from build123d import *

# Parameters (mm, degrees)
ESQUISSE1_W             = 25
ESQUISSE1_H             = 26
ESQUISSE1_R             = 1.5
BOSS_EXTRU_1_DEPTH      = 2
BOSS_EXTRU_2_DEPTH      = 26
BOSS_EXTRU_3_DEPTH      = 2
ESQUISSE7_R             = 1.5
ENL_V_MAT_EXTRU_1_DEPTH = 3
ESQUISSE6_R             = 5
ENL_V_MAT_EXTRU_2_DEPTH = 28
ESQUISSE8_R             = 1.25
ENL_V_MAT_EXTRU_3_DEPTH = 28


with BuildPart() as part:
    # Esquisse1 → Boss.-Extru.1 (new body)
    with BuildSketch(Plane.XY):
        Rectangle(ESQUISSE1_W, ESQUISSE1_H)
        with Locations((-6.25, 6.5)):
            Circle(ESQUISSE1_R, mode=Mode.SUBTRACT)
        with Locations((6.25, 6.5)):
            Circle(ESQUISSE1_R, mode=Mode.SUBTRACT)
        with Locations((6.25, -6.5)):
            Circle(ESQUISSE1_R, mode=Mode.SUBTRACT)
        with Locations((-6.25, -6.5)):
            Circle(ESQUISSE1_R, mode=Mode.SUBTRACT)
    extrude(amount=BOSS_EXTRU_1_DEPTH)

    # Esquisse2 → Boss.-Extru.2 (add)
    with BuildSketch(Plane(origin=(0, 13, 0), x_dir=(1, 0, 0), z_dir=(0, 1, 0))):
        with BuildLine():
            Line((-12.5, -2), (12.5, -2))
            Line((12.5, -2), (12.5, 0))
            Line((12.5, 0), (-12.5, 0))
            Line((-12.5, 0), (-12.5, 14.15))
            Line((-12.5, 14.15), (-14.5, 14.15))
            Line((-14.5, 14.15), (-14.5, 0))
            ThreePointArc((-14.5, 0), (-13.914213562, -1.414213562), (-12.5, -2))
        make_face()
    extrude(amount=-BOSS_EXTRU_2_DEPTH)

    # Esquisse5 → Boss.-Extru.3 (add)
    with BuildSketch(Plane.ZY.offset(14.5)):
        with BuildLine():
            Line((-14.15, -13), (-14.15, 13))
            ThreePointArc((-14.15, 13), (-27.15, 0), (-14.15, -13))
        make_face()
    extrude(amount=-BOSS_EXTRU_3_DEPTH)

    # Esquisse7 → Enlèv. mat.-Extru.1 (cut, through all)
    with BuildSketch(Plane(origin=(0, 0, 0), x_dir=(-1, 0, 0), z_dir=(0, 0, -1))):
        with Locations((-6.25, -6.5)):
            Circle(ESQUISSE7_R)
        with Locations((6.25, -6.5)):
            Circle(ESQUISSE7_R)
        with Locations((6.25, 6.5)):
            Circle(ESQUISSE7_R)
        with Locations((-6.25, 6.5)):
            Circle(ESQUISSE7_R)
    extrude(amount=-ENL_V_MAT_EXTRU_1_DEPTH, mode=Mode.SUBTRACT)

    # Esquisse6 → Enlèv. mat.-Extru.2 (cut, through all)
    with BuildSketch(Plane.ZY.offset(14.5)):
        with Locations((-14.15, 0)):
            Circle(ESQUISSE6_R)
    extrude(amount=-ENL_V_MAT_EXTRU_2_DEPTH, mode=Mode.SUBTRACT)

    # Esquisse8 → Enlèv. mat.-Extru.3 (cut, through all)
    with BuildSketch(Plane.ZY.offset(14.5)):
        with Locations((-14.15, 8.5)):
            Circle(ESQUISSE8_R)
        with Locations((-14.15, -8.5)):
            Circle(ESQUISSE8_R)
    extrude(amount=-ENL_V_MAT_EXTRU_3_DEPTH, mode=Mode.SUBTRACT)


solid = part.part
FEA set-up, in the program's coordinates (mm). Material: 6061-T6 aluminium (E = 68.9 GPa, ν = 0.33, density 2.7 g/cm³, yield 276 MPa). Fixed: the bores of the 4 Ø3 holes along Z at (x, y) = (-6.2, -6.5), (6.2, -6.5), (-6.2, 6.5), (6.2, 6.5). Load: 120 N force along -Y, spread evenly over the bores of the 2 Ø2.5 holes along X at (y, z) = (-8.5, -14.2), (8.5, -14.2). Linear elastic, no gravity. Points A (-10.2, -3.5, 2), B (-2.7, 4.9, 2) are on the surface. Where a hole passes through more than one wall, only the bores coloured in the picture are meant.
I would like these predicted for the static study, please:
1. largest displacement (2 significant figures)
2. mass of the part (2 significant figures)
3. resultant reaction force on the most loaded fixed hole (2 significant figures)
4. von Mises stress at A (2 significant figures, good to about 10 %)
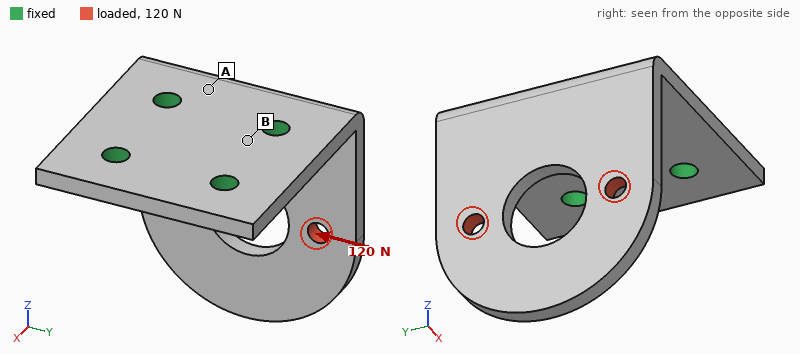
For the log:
55 µm
6.5 g
140 N
23 MPa
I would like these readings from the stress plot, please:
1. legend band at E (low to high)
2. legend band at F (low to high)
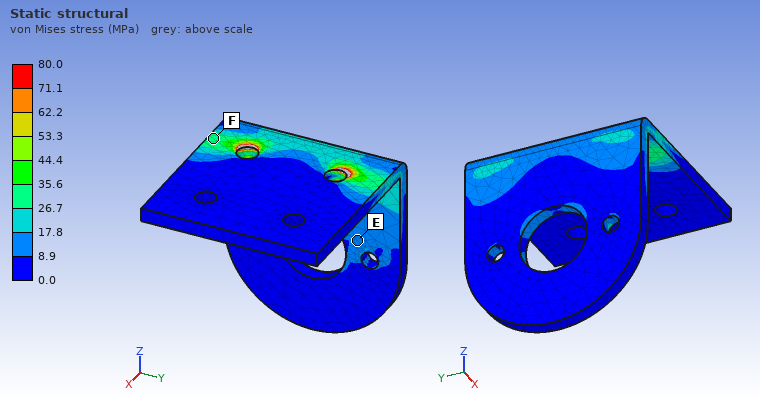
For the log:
8.9 to 17.8 MPa
26.7 to 35.6 MPa
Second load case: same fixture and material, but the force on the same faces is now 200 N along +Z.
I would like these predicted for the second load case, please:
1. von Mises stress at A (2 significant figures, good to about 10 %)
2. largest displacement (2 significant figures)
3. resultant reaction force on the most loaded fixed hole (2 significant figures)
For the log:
34 MPa
0.11 mm
110 N
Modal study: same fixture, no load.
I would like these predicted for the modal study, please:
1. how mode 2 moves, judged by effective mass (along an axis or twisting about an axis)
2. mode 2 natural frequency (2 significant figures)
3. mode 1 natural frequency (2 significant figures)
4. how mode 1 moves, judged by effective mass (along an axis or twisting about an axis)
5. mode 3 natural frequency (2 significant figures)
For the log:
along Y
4800 Hz
1800 Hz
along X
6700 Hz
